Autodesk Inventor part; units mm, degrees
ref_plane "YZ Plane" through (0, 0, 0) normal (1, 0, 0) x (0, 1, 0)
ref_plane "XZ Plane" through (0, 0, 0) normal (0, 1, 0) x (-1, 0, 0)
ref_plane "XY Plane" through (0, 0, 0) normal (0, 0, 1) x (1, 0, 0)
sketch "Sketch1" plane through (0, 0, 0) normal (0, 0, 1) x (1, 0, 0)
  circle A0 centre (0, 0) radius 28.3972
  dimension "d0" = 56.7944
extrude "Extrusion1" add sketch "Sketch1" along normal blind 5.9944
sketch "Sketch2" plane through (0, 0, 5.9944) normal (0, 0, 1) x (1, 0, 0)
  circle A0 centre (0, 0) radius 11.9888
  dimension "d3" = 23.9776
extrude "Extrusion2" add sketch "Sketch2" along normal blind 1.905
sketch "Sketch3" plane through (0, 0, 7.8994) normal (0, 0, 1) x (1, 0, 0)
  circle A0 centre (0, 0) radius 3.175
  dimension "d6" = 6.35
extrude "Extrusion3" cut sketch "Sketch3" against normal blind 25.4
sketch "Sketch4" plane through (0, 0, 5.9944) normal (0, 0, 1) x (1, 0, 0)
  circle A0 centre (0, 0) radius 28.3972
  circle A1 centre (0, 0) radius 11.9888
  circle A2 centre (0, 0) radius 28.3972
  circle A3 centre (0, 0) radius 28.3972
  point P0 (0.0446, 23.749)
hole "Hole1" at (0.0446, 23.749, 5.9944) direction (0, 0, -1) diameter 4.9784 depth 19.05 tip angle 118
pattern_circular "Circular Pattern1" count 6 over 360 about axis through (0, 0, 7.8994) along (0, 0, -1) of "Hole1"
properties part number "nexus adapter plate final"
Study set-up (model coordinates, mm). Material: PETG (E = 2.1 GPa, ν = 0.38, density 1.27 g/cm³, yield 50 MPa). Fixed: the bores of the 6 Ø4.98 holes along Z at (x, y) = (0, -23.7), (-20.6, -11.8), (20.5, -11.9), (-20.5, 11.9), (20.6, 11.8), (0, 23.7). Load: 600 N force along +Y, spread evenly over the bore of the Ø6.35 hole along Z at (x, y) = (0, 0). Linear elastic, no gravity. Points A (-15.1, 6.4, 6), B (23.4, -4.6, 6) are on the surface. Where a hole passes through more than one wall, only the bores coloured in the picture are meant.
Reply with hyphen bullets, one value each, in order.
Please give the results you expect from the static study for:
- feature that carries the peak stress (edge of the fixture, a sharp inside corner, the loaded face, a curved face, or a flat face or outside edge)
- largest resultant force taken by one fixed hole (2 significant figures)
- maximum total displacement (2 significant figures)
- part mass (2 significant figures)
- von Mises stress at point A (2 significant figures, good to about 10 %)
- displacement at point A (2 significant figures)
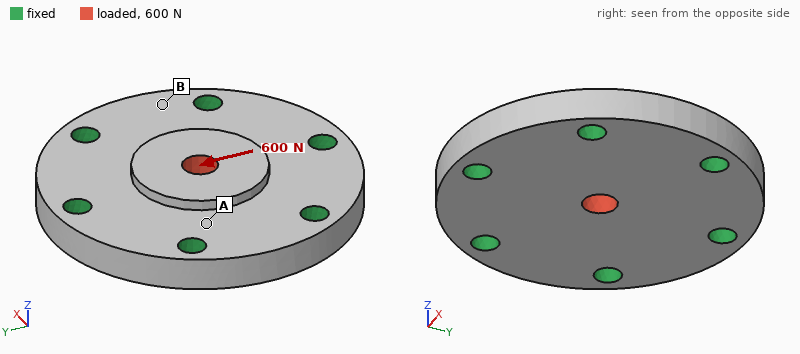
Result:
- the loaded face
- 160 N
- 27 µm
- 19 g
- 1.3 MPa
- 4.0 µm
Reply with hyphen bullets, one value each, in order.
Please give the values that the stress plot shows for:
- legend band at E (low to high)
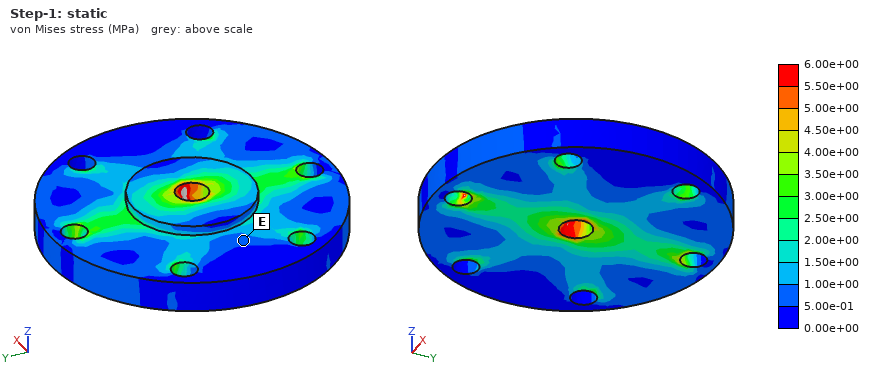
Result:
- 5.00e-01 to 1.00e+00 MPa
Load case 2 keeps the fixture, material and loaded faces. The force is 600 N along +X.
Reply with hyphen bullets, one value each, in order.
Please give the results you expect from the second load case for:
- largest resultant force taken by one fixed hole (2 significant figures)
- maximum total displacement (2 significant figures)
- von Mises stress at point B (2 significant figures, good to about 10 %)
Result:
- 140 N
- 27 µm
- 0.71 MPa
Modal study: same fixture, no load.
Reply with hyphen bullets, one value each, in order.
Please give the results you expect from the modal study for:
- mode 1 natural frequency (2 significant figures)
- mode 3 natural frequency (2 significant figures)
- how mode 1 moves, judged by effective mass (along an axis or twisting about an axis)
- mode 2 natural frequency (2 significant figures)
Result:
- 5600 Hz
- 9900 Hz
- along Z
- 9900 Hz
